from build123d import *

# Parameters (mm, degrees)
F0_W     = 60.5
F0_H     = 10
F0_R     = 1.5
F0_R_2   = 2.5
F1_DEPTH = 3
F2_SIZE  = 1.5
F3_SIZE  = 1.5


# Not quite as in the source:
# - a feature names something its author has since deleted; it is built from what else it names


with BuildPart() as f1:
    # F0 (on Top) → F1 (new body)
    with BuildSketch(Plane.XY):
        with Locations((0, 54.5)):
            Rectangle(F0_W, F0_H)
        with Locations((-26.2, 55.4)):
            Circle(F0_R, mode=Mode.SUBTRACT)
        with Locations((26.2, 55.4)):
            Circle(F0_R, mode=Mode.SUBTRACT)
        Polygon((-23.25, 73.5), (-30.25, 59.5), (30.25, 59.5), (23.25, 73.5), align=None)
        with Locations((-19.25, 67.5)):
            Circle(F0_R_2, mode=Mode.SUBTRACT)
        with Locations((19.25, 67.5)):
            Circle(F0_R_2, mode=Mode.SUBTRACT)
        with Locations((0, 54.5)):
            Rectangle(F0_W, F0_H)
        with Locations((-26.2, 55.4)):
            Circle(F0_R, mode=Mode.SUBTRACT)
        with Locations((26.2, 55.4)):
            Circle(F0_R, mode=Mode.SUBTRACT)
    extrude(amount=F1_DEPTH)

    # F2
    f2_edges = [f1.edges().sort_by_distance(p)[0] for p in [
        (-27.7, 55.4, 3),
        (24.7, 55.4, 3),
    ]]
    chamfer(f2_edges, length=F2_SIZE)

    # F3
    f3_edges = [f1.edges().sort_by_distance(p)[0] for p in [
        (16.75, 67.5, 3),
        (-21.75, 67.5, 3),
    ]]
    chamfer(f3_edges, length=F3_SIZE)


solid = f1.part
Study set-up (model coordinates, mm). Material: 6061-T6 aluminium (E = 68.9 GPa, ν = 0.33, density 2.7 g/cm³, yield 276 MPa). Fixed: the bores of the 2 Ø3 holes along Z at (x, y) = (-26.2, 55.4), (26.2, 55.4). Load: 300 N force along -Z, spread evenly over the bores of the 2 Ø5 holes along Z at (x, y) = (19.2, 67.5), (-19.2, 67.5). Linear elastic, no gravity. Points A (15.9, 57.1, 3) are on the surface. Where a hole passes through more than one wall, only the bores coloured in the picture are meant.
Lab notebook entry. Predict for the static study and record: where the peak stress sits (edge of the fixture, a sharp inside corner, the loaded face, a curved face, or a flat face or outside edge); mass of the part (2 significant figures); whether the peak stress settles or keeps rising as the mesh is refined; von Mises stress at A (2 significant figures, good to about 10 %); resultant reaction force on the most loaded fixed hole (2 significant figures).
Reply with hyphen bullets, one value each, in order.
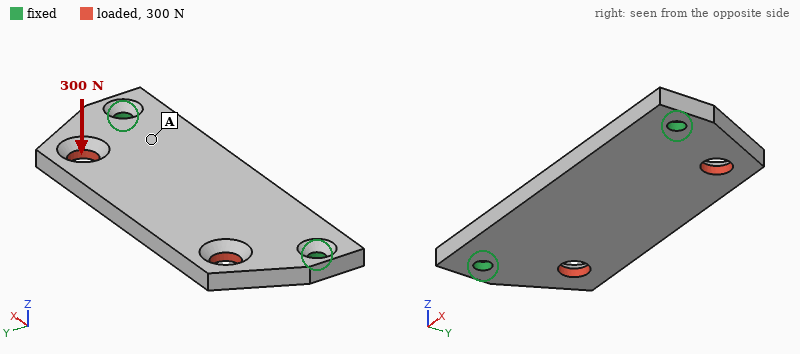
- edge of the fixture
- 10 g
- keeps rising
- 32 MPa
- 170 N
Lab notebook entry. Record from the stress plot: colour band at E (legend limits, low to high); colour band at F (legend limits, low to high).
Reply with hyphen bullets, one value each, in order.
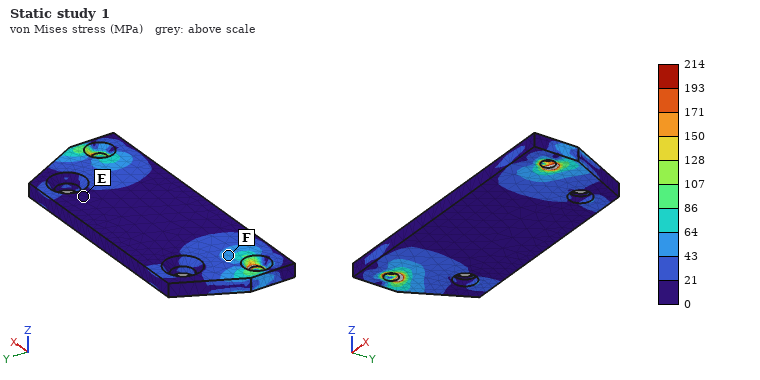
- 0 to 21 MPa
- 43 to 64 MPa
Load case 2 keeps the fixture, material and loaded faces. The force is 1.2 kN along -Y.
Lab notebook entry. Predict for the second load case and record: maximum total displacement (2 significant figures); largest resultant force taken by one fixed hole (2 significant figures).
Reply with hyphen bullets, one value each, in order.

- 27 µm
- 630 N
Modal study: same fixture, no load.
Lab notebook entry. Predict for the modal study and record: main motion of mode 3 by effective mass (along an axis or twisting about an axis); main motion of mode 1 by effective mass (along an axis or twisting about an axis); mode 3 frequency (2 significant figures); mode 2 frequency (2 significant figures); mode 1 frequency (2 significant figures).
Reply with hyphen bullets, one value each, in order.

- twisting about Y
- along Z
- 8000 Hz
- 6000 Hz
- 3200 Hz
